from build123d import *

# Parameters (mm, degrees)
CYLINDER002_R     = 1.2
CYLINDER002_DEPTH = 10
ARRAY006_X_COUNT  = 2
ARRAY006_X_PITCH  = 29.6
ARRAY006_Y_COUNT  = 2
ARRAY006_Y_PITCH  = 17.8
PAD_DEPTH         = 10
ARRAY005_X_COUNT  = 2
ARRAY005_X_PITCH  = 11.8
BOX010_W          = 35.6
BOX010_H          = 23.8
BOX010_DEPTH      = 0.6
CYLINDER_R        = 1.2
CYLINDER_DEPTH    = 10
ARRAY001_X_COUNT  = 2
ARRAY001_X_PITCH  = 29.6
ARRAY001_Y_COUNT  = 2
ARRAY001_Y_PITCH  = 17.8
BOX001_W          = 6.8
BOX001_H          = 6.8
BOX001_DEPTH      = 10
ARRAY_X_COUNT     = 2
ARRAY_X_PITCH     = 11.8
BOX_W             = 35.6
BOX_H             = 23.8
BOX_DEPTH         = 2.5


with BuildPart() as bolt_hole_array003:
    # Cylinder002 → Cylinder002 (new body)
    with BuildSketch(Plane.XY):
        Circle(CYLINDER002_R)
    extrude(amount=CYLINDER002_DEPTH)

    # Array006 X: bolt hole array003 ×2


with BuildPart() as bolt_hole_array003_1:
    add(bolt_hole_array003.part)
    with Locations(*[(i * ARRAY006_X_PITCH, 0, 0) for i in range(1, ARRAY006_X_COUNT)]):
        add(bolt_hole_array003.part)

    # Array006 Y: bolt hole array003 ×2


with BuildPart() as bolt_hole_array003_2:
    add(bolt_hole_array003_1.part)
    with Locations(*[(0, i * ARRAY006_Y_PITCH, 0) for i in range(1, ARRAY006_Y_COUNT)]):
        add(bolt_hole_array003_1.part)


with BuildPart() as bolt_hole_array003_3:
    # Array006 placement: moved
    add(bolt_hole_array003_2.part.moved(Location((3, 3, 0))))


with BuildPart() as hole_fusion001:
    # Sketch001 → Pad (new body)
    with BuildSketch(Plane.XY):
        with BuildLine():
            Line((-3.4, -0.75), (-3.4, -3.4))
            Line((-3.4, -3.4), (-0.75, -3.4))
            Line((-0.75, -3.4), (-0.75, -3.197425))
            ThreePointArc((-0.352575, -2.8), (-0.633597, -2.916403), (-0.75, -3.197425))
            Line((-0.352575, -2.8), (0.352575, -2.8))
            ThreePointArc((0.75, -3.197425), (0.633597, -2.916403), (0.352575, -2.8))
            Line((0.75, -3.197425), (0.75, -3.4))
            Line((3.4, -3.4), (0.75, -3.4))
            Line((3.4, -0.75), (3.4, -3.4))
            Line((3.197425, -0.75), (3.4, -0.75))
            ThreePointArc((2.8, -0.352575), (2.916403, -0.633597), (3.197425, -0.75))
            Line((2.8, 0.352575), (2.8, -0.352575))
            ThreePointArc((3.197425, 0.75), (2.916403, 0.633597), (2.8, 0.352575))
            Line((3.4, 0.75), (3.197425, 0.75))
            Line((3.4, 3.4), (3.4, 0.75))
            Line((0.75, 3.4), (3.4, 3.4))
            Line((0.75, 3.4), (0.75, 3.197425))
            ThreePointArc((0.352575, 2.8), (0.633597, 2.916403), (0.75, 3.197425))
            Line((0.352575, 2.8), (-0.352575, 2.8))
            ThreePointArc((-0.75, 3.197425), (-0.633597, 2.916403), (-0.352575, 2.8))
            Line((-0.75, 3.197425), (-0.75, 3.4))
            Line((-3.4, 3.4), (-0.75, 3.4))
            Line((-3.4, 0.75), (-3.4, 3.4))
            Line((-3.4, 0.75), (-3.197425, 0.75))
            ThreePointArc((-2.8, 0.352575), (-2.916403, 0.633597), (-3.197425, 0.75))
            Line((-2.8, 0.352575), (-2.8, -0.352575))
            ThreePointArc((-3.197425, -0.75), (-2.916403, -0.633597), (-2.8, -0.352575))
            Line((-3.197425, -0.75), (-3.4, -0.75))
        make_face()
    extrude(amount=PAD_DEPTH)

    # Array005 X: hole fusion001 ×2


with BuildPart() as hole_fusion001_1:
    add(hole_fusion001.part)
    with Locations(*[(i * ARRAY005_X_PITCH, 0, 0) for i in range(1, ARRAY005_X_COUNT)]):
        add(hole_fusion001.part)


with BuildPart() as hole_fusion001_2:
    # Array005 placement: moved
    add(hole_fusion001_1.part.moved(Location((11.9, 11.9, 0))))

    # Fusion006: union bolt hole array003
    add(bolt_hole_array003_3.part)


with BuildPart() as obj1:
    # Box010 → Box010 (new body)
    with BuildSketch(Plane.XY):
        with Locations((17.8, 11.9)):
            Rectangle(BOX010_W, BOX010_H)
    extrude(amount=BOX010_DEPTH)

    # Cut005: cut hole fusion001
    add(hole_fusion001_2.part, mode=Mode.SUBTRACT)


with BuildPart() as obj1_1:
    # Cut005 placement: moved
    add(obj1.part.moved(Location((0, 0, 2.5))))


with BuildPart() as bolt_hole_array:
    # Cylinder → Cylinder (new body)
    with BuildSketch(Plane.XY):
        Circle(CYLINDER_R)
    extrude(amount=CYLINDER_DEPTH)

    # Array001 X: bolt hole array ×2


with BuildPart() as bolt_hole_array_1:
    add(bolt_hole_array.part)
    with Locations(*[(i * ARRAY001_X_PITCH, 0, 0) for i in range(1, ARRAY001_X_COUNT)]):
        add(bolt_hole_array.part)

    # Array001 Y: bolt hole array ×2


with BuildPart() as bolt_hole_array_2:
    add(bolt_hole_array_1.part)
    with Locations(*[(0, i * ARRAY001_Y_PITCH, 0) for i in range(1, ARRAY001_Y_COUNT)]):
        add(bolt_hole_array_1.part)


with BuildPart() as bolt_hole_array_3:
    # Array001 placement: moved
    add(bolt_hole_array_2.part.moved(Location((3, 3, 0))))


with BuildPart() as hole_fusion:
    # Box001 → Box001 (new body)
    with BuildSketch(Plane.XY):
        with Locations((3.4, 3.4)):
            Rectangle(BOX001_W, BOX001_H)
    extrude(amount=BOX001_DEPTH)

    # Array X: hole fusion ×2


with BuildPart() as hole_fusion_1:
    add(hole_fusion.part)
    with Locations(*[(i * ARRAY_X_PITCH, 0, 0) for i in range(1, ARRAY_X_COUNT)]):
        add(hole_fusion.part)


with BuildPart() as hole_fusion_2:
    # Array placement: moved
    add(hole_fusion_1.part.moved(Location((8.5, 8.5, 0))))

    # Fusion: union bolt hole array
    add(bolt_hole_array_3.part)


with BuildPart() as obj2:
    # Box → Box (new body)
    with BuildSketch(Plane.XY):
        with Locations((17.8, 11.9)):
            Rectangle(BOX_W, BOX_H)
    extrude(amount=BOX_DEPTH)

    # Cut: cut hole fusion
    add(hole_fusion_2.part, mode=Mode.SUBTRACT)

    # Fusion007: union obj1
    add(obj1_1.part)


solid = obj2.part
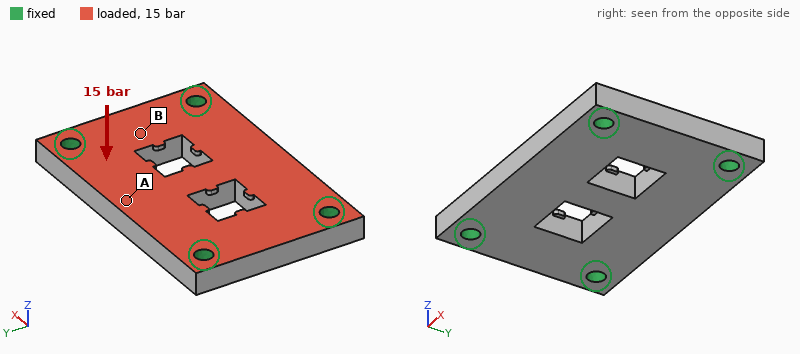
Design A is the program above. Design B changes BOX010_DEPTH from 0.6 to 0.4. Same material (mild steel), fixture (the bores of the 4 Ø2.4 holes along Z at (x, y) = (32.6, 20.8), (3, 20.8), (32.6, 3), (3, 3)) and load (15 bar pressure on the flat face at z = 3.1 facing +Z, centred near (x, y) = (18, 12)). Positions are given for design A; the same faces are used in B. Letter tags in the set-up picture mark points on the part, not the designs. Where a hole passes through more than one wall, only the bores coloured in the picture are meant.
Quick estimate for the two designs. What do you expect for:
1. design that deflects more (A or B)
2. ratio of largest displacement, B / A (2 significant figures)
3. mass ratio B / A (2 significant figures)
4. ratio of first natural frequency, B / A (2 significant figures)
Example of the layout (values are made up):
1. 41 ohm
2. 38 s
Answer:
1. B
2. 1.2
3. 0.94
4. 0.95
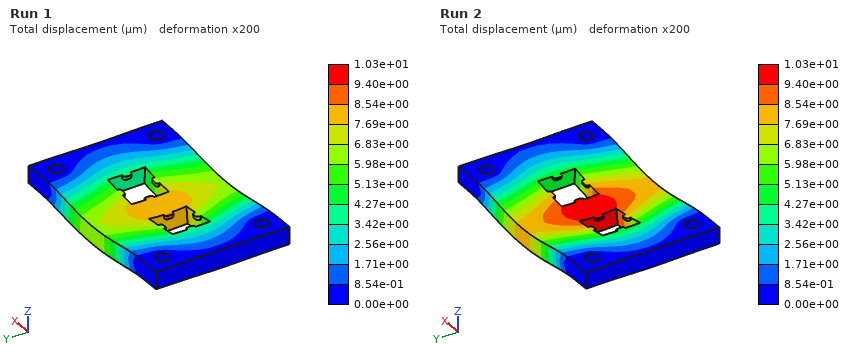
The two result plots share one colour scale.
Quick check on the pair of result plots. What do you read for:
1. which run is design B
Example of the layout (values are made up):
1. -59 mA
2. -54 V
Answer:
1. Run 2
